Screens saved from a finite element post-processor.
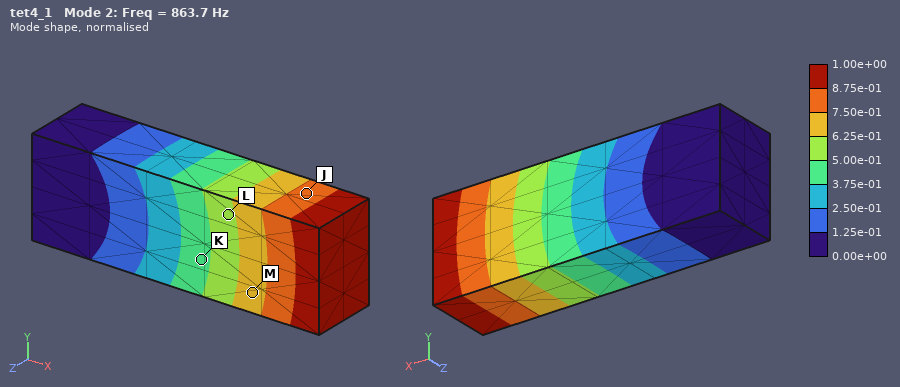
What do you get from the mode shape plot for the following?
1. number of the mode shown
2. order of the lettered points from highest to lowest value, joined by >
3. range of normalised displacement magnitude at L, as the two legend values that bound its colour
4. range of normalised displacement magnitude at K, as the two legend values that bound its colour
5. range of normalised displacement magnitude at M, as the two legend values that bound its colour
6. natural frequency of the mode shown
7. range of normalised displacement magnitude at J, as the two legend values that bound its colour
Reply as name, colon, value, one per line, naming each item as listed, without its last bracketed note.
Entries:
number of the mode shown: 2
order of the lettered points from highest to lowest value, joined by >: J > M > L > K
range of normalised displacement magnitude at L, as the two legend values that bound its colour: 5.00e-01 to 6.25e-01
range of normalised displacement magnitude at K, as the two legend values that bound its colour: 3.75e-01 to 5.00e-01
range of normalised displacement magnitude at M, as the two legend values that bound its colour: 6.25e-01 to 7.50e-01
natural frequency of the mode shown: 863.7 Hz
range of normalised displacement magnitude at J, as the two legend values that bound its colour: 7.50e-01 to 8.75e-01
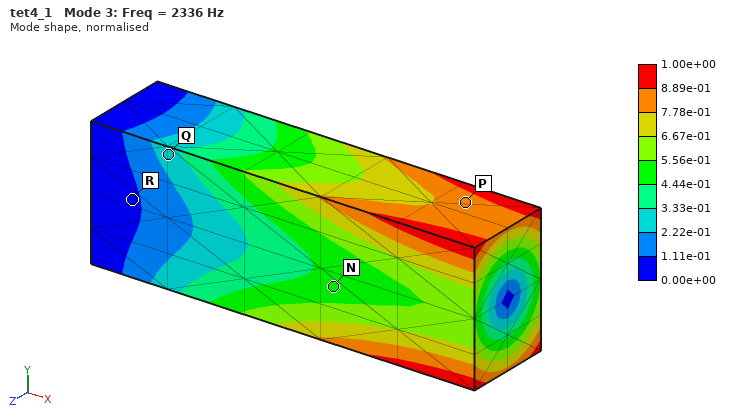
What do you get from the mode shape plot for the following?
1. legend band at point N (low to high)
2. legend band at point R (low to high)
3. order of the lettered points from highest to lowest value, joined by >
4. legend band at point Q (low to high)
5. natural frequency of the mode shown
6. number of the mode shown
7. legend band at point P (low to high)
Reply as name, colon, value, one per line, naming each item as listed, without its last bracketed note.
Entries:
legend band at point N: 4.44e-01 to 5.56e-01
legend band at point R: 0.00e+00 to 1.11e-01
order of the lettered points from highest to lowest value, joined by >: P > N > Q > R
legend band at point Q: 2.22e-01 to 3.33e-01
natural frequency of the mode shown: 2336 Hz
number of the mode shown: 3
legend band at point P: 7.78e-01 to 8.89e-01
